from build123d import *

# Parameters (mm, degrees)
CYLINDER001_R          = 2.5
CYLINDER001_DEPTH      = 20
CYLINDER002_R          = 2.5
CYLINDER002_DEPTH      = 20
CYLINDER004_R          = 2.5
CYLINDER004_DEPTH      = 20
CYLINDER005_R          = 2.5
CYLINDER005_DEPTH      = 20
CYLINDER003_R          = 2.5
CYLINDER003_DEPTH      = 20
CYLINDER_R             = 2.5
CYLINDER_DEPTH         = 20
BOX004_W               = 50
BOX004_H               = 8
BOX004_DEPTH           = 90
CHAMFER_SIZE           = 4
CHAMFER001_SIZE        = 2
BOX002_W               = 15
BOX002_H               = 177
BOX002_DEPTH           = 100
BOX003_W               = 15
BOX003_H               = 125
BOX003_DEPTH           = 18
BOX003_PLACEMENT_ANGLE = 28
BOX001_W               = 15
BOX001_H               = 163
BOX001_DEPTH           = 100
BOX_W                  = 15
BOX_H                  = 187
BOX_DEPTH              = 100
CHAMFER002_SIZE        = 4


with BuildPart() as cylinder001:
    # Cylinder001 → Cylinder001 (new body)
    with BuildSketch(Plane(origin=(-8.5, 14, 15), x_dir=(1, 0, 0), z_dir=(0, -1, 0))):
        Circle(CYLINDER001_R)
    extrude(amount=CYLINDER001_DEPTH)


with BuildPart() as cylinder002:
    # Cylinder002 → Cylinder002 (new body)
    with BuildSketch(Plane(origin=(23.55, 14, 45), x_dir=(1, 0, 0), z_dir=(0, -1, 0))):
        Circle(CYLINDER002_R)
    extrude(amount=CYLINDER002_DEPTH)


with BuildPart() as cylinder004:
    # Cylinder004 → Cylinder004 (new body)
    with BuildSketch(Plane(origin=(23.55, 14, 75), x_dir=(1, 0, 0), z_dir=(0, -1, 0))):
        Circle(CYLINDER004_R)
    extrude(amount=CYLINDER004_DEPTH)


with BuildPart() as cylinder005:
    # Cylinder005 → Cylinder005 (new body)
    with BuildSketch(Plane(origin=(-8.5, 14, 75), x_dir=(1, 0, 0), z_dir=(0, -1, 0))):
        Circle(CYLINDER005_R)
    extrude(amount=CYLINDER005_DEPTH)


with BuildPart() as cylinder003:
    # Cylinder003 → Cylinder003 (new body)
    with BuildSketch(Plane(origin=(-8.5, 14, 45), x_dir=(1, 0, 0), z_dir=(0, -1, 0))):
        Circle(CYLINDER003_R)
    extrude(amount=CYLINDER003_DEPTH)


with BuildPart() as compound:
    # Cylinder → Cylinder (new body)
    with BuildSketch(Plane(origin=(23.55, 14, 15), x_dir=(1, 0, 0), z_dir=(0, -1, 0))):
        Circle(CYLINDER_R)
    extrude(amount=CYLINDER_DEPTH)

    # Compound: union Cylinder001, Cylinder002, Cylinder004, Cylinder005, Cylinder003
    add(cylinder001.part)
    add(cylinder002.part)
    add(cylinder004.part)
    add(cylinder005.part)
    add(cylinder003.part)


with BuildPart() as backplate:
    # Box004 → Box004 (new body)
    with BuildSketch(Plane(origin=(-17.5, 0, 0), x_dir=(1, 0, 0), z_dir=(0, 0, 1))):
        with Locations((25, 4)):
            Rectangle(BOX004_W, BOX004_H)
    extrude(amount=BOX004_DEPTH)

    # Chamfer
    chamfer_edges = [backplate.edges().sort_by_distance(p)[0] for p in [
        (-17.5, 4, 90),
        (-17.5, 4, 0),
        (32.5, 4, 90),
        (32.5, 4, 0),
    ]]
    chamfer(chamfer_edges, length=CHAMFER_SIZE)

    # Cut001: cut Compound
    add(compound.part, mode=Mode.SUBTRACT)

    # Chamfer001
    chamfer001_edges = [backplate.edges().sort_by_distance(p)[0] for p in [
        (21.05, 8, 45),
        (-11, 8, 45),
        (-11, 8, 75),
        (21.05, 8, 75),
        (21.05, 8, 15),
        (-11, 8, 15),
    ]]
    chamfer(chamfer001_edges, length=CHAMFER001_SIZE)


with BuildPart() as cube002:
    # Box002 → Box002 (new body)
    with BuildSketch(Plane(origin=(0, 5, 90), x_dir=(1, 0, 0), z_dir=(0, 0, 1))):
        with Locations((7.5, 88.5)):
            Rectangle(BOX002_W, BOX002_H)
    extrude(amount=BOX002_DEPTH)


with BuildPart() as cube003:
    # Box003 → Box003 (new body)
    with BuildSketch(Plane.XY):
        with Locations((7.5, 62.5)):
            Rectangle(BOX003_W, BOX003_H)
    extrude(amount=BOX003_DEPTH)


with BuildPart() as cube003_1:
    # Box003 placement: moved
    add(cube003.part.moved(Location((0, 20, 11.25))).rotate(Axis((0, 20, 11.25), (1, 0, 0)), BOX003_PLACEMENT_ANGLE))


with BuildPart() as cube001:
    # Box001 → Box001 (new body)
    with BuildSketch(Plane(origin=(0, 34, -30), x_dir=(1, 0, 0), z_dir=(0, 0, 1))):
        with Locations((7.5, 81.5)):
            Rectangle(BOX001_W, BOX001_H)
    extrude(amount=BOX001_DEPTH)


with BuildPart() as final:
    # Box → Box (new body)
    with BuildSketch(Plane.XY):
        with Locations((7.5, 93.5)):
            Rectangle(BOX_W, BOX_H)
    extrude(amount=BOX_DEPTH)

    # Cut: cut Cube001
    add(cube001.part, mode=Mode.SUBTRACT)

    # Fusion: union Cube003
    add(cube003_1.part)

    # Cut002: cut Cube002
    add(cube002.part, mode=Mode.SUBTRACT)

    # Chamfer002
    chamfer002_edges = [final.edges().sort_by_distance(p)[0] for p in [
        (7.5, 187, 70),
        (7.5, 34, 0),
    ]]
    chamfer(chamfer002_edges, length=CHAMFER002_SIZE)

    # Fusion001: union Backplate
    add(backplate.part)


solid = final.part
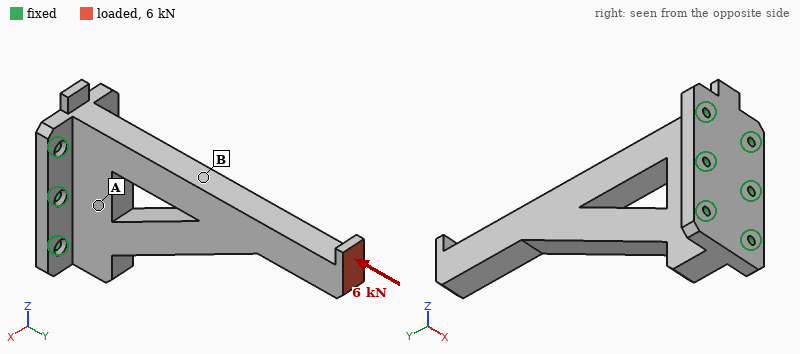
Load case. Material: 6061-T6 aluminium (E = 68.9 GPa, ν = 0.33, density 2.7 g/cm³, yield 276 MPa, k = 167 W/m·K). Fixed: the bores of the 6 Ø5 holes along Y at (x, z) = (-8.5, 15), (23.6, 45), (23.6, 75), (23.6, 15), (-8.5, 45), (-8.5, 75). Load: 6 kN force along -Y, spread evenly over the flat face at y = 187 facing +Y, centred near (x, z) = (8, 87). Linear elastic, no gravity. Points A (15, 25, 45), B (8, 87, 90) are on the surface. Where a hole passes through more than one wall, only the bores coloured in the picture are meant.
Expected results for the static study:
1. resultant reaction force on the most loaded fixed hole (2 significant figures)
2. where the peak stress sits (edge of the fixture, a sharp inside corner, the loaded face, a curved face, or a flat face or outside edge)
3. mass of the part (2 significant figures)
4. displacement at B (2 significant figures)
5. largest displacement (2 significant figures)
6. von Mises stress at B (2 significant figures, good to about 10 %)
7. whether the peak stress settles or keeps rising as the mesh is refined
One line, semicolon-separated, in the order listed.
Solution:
3.4 kN; edge of the fixture; 380 g; 0.077 mm; 0.47 mm; 39 MPa; keeps rising
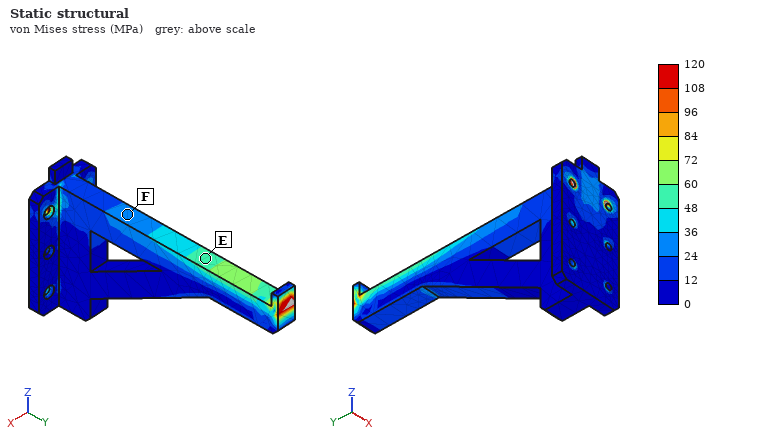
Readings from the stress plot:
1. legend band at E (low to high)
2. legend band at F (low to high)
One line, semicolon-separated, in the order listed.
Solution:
48 to 60 MPa; 24 to 36 MPa
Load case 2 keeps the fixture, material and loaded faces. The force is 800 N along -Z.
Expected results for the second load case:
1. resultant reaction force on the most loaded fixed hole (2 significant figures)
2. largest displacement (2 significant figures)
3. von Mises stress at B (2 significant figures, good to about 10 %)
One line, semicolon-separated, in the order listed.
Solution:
1.3 kN; 0.32 mm; 22 MPa
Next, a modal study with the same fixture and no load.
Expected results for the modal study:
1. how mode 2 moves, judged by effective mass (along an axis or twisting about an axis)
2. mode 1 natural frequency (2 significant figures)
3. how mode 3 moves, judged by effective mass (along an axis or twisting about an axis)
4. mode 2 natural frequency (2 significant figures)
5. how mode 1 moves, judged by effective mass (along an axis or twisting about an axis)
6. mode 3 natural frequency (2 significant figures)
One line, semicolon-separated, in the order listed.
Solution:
along Z; 490 Hz; along X; 1600 Hz; along X; 2300 Hz
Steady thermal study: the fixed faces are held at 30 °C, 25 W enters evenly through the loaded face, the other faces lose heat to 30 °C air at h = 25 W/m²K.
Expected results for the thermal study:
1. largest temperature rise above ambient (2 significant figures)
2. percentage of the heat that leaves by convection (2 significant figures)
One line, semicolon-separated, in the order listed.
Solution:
58 K; 34 %
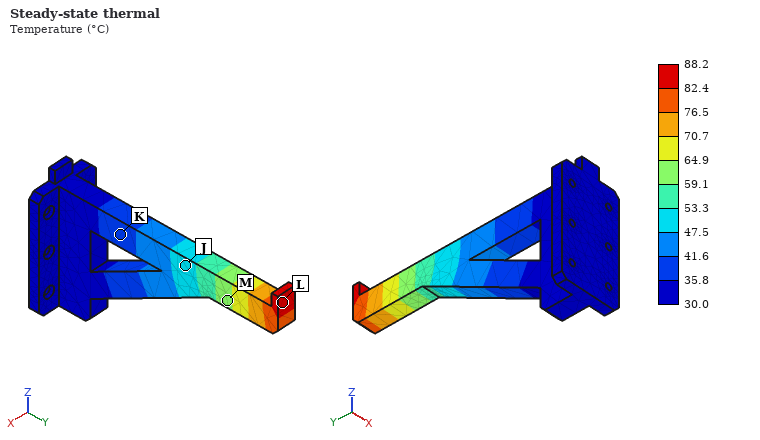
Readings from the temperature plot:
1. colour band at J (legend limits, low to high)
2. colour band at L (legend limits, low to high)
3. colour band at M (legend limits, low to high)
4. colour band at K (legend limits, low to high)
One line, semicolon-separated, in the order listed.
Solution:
47.5 to 53.3 °C; 82.4 to 88.2 °C; 59.1 to 64.9 °C; 35.8 to 41.6 °C
